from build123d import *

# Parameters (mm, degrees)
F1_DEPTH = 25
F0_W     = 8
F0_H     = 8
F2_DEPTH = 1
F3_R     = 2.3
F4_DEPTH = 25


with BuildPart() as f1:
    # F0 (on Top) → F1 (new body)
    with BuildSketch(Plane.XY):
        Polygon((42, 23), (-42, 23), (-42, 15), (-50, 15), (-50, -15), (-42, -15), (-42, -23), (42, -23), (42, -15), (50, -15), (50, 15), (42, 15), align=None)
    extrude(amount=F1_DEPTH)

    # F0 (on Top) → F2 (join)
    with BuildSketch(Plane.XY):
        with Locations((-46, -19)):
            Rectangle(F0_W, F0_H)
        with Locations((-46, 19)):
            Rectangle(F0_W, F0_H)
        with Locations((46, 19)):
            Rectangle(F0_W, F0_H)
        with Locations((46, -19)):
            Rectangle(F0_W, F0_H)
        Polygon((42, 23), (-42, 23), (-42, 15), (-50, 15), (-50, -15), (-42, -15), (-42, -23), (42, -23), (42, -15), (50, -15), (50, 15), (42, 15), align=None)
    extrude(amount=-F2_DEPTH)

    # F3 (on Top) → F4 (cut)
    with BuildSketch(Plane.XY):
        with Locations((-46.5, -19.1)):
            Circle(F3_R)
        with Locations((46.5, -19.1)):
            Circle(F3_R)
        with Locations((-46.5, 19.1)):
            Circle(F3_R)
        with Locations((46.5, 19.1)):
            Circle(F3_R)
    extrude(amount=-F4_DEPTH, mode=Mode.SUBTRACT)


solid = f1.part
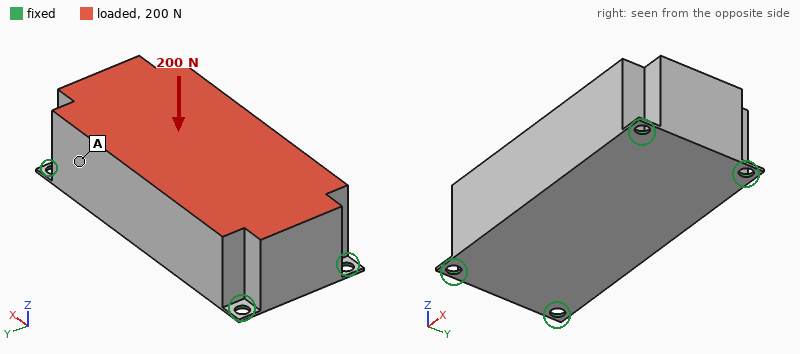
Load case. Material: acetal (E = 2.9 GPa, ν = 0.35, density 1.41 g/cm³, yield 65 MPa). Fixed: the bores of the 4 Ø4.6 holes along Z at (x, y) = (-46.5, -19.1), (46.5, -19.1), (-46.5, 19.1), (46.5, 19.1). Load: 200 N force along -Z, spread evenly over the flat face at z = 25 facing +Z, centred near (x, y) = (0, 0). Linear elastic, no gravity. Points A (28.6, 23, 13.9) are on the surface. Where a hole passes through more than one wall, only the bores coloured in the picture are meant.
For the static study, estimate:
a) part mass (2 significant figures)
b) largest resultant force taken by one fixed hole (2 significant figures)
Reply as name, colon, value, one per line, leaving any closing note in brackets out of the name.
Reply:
part mass: 160 g
largest resultant force taken by one fixed hole: 59 N
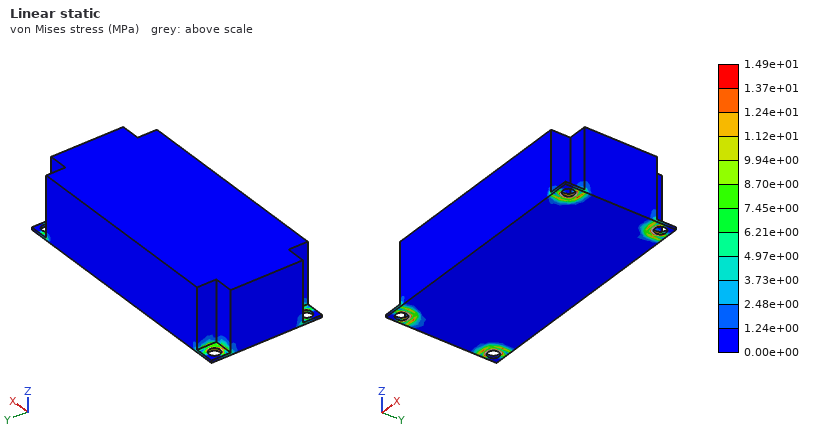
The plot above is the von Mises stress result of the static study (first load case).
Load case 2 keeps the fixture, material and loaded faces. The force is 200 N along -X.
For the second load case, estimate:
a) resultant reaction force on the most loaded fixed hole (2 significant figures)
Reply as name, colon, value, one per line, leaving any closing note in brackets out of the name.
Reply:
resultant reaction force on the most loaded fixed hole: 60 N
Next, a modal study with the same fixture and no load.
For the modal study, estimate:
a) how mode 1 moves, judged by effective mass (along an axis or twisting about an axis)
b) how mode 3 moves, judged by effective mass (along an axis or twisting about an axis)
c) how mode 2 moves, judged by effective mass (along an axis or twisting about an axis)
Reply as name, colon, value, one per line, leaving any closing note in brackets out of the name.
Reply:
how mode 1 moves, judged by effective mass: along Y
how mode 3 moves, judged by effective mass: along X
how mode 2 moves, judged by effective mass: along Z
